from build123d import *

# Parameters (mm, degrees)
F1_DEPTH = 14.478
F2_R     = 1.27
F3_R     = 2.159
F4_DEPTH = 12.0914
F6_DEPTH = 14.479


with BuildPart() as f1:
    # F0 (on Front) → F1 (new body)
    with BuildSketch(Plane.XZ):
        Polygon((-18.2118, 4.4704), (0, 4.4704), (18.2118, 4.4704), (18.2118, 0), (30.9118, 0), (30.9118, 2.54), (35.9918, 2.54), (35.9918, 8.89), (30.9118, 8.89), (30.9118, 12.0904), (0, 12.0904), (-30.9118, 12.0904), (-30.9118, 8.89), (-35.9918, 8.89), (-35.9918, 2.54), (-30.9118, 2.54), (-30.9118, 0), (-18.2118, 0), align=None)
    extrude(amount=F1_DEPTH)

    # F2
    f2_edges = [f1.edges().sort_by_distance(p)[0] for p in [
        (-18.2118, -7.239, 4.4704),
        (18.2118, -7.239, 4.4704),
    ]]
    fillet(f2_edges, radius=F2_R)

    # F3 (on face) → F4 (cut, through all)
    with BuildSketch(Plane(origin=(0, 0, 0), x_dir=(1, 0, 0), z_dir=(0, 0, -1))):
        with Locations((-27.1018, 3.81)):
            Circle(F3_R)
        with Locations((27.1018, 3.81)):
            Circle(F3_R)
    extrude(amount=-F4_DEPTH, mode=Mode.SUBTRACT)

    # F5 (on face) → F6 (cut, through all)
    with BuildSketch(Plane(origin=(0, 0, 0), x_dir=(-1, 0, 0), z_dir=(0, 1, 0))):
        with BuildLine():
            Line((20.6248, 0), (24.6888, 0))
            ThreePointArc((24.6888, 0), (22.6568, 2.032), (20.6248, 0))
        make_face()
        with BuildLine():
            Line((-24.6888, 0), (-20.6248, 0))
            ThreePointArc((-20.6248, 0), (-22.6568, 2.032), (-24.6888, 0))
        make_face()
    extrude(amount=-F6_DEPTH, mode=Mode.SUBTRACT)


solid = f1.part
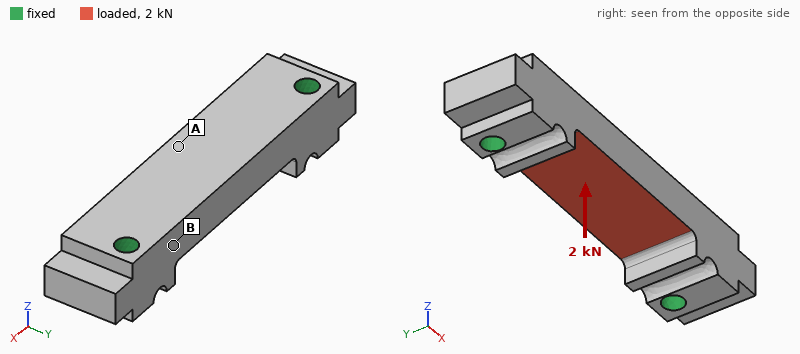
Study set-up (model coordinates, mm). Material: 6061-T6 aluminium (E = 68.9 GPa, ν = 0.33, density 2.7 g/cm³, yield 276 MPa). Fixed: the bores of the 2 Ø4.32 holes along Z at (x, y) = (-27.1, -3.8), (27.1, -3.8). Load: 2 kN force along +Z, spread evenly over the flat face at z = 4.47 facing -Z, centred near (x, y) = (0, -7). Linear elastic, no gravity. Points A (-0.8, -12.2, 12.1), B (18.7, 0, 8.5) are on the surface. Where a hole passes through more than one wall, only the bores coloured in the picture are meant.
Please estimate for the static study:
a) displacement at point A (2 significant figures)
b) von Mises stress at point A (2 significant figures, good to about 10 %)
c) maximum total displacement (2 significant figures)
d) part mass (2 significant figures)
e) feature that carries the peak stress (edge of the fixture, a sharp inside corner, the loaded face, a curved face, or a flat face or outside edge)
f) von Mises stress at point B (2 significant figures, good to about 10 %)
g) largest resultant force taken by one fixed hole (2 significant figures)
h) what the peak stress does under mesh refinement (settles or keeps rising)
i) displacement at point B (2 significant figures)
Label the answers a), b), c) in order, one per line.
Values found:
a) 28 µm
b) 40 MPa
c) 29 µm
d) 24 g
e) edge of the fixture
f) 16 MPa
g) 1.0 kN
h) keeps rising
i) 4.9 µm
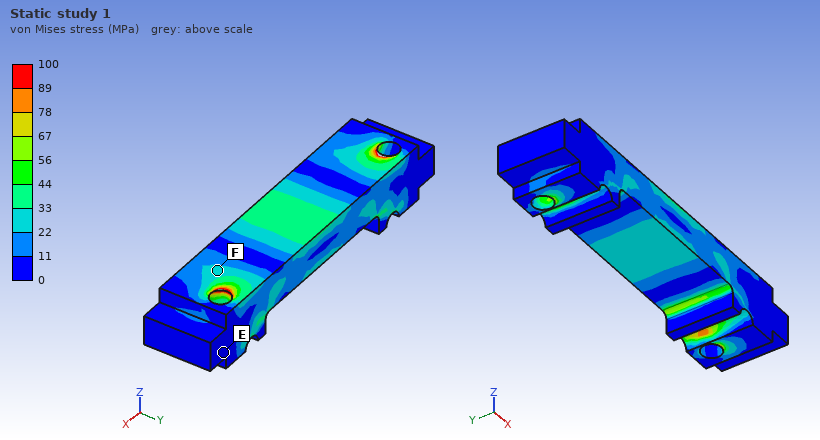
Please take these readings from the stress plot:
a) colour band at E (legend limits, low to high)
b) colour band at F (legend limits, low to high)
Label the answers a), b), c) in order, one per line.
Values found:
a) 0 to 11 MPa
b) 22 to 33 MPa
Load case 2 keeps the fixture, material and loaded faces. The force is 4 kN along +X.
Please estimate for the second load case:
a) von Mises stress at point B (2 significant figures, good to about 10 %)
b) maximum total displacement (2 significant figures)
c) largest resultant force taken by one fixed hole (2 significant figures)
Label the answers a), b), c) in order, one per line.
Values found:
a) 27 MPa
b) 7.8 µm
c) 2.0 kN
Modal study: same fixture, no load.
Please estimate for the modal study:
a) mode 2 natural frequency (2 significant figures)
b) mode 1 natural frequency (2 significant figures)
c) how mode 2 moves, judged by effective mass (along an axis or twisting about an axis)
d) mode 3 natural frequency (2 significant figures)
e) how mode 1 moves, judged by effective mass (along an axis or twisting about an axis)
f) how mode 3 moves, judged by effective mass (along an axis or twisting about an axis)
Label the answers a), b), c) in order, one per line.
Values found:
a) 16 kHz
b) 15 kHz
c) along Y
d) 26 kHz
e) along Z
f) twisting about X
